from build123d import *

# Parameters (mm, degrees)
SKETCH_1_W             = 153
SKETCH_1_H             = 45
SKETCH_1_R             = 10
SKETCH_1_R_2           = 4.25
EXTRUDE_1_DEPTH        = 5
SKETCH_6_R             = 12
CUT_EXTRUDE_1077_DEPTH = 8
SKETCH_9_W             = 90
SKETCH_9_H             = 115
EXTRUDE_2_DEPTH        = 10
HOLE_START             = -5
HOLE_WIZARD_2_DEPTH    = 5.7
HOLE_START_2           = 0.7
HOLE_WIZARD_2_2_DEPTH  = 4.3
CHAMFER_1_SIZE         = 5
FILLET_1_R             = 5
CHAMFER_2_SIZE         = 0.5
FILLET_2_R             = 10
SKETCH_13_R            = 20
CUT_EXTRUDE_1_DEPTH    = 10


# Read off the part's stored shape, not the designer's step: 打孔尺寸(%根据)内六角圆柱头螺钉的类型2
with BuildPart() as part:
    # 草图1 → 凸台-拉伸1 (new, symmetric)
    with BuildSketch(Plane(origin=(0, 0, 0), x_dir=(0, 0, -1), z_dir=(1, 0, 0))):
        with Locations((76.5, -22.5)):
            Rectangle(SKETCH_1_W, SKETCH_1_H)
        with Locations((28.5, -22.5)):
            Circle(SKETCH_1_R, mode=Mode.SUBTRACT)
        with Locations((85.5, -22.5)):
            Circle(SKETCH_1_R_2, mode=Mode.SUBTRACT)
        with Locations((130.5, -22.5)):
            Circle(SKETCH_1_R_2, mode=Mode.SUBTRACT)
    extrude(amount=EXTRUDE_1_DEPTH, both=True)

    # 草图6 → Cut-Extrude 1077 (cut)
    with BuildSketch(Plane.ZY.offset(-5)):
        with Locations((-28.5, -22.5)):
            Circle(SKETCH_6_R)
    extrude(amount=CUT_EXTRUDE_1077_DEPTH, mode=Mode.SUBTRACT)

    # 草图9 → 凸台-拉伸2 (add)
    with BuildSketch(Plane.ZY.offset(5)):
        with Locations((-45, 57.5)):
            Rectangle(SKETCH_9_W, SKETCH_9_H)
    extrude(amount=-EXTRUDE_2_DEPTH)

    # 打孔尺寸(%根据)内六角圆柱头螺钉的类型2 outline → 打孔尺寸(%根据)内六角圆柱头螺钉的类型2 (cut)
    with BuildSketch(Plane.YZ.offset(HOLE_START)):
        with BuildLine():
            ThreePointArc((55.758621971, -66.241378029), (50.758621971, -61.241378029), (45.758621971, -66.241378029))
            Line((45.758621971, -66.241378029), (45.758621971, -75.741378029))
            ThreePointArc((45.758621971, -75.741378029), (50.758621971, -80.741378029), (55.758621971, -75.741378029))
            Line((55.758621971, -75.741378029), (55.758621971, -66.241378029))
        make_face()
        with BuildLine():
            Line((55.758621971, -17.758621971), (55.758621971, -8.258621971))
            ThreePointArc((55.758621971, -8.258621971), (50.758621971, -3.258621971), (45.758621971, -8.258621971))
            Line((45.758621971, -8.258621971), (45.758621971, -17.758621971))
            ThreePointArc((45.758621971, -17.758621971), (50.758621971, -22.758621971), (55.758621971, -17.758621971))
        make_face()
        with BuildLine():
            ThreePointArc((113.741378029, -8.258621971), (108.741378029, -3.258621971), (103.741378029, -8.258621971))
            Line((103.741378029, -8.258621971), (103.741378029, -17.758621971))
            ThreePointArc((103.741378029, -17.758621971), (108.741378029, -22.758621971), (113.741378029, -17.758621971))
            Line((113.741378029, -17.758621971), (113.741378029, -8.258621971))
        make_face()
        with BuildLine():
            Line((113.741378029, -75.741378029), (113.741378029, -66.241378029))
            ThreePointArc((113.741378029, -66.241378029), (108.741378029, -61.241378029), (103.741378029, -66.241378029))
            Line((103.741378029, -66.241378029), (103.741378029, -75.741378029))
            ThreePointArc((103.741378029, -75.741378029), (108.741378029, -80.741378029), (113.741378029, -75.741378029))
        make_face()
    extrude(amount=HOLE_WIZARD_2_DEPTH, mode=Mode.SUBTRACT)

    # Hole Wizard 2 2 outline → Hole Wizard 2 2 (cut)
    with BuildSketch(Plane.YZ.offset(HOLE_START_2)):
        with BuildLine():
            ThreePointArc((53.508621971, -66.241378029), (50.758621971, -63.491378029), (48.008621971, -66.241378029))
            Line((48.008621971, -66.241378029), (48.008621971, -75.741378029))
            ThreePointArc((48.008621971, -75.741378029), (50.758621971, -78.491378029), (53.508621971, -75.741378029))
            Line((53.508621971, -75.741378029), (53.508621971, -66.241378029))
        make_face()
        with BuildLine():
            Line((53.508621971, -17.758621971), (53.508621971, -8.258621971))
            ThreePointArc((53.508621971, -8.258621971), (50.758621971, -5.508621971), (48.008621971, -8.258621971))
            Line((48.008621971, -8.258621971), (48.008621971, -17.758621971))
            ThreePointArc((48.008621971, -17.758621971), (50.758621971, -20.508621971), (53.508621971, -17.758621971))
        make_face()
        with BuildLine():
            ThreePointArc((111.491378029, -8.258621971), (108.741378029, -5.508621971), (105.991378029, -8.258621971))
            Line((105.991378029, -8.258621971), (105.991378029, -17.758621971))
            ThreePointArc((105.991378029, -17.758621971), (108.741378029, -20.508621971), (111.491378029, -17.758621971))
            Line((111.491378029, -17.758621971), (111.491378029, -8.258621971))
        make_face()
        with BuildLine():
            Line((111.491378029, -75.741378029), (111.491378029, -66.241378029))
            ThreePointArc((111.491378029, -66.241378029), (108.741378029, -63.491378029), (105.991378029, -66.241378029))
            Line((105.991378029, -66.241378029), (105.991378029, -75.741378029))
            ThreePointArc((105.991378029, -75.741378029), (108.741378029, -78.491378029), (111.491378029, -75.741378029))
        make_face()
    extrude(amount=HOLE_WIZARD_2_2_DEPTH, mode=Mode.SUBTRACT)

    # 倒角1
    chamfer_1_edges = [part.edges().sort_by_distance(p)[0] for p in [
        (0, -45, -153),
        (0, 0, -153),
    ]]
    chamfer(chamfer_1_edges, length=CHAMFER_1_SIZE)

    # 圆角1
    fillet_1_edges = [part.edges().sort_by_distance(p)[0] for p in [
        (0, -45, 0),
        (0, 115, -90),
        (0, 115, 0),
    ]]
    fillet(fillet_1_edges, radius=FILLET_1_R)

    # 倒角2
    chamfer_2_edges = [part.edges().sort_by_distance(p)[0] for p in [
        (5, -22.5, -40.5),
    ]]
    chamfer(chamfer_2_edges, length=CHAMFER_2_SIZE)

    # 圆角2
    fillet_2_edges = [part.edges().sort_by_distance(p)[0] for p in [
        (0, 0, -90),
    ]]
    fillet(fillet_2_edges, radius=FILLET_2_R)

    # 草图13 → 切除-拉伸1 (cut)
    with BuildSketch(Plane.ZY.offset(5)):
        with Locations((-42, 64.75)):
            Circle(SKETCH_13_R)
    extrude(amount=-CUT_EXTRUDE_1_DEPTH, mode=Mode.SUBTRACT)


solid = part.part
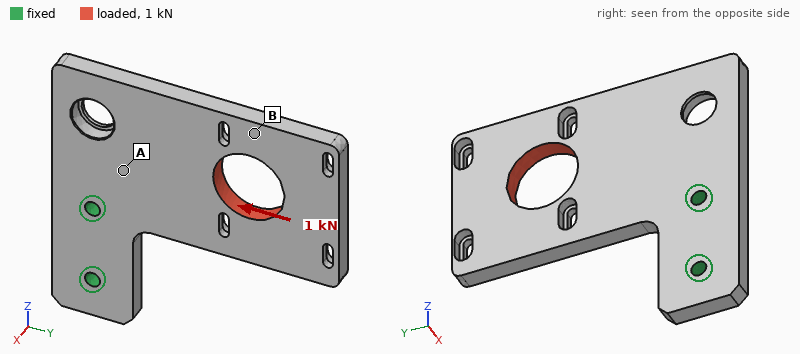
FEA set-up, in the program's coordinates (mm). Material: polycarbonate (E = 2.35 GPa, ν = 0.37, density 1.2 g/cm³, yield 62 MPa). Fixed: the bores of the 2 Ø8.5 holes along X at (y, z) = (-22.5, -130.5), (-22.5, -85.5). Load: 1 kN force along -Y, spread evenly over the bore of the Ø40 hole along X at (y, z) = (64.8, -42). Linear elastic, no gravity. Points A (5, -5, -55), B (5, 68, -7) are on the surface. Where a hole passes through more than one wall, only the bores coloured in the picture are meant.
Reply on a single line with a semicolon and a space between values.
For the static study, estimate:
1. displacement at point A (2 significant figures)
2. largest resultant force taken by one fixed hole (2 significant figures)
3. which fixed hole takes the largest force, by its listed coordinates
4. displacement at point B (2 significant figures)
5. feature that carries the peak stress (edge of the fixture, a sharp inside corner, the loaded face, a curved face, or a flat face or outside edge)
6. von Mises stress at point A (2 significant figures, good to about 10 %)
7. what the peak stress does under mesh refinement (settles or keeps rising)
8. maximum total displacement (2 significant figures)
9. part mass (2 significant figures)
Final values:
0.31 mm; 1.7 kN; (-22.5, -85.5); 1.1 mm; edge of the fixture; 3.0 MPa; keeps rising; 1.5 mm; 180 g
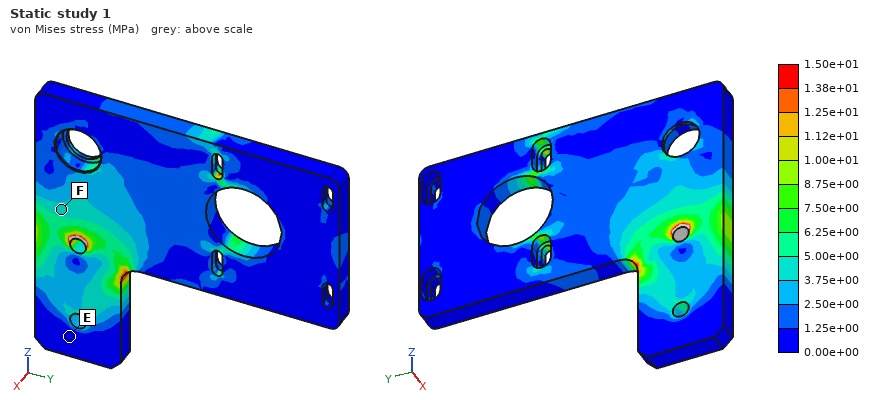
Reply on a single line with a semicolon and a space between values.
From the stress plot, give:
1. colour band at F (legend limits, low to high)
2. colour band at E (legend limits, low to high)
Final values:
3.75e+00 to 5.00e+00 MPa; 0.00e+00 to 1.25e+00 MPa
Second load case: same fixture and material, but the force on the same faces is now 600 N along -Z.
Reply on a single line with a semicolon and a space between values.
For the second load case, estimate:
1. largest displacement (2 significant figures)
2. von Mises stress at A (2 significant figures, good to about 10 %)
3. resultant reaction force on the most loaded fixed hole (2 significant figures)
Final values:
1.9 mm; 2.7 MPa; 970 N
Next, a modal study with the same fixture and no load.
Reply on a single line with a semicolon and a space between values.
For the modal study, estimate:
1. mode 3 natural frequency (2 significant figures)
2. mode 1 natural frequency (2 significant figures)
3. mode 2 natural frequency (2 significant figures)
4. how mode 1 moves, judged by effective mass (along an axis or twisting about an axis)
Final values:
330 Hz; 95 Hz; 230 Hz; along X
